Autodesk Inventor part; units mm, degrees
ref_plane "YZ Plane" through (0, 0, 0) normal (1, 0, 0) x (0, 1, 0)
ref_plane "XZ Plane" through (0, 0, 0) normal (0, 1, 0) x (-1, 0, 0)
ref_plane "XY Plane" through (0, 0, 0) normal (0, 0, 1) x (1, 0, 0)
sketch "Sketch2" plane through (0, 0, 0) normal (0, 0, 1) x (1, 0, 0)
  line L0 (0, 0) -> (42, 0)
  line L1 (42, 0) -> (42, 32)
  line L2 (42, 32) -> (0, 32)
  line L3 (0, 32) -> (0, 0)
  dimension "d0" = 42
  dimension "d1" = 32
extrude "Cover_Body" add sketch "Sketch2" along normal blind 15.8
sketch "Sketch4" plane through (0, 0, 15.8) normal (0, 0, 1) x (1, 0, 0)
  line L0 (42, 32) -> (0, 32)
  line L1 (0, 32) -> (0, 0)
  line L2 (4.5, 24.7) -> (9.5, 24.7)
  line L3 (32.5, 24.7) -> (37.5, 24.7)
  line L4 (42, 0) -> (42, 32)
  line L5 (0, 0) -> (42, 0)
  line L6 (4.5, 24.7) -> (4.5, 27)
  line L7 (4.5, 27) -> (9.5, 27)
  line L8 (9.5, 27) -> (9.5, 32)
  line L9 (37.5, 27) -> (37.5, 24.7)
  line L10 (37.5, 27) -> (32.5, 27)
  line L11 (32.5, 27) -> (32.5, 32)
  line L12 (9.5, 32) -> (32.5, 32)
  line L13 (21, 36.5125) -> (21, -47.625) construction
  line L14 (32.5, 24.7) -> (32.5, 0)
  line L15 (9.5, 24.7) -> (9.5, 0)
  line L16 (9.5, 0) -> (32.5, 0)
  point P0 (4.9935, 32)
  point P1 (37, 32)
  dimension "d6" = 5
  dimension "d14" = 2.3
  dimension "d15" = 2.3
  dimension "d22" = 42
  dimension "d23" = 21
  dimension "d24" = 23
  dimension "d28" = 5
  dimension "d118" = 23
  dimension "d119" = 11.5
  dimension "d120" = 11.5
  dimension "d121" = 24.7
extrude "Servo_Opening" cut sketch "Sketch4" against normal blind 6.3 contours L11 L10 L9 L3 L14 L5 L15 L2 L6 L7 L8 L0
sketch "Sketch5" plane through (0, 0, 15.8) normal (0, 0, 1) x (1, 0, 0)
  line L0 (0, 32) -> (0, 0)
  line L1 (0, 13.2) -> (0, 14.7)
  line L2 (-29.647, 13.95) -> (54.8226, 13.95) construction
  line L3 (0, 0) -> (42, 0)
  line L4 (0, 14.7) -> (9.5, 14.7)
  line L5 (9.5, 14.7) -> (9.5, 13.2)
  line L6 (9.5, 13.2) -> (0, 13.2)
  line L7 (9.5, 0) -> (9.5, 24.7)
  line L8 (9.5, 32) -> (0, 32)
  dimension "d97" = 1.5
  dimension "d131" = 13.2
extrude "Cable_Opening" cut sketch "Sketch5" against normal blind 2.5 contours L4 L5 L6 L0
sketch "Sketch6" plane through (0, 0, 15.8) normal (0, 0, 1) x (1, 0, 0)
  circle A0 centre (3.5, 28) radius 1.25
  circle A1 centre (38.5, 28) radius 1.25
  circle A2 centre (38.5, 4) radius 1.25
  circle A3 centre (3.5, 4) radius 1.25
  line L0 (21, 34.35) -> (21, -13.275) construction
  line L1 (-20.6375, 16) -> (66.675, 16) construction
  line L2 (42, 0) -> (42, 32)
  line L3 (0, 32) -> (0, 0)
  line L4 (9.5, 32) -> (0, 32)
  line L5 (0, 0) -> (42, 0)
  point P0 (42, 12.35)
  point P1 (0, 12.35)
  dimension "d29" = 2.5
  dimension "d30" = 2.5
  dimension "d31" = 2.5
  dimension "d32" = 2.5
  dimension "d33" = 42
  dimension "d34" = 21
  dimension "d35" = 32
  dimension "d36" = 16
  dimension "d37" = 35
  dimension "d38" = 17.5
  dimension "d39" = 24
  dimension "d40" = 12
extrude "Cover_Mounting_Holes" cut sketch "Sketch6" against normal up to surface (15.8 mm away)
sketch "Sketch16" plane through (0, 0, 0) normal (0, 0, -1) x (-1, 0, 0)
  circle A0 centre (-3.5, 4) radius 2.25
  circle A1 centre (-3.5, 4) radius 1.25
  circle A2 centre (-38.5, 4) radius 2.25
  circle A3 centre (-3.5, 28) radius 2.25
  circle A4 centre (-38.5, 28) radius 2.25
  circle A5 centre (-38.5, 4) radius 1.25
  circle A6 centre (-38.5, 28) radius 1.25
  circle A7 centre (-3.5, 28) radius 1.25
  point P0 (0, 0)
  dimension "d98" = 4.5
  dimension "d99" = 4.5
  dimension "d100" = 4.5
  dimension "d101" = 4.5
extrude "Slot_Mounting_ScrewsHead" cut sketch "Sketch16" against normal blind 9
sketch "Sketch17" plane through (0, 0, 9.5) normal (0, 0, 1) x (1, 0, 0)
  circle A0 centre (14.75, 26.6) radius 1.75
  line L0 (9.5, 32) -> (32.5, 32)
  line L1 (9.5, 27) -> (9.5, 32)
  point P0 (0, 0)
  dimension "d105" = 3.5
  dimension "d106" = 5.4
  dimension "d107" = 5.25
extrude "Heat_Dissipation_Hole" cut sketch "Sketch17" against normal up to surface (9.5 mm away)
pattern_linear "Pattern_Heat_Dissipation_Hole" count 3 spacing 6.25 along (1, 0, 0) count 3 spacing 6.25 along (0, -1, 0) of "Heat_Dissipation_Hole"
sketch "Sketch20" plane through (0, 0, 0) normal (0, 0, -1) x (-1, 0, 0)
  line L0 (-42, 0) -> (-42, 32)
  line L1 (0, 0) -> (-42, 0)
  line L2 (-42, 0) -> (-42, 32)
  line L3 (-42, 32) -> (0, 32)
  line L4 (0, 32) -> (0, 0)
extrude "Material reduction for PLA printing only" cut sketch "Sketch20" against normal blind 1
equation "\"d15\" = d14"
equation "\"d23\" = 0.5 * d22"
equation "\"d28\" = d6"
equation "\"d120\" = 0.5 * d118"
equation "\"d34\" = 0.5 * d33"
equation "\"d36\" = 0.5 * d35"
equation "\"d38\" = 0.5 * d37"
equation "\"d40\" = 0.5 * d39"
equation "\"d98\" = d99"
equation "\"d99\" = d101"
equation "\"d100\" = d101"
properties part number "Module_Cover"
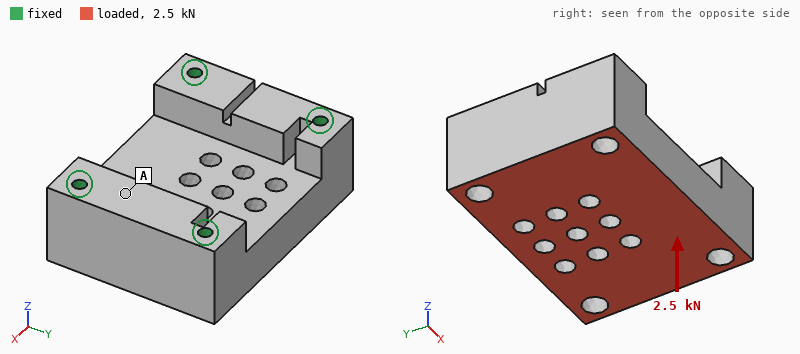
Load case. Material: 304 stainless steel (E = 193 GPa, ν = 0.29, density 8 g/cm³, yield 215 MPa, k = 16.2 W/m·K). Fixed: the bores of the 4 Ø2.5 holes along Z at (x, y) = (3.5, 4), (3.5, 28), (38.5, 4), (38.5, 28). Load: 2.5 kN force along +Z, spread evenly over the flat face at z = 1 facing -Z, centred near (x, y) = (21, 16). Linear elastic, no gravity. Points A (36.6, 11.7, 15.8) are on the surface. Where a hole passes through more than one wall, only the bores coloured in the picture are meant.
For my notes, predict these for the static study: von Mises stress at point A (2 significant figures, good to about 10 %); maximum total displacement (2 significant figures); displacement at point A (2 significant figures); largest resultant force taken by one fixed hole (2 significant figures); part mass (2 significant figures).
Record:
4.0 MPa
1.9 µm
0.81 µm
770 N
110 g
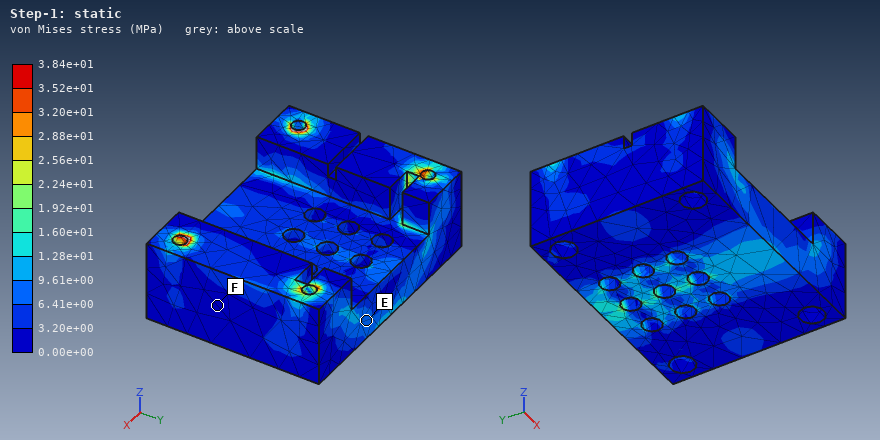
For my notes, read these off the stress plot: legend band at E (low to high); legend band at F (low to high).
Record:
6.41e+00 to 9.61e+00 MPa
0.00e+00 to 3.20e+00 MPa
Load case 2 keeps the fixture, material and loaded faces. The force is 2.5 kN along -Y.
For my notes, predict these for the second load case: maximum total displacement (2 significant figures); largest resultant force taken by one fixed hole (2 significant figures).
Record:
2.2 µm
880 N
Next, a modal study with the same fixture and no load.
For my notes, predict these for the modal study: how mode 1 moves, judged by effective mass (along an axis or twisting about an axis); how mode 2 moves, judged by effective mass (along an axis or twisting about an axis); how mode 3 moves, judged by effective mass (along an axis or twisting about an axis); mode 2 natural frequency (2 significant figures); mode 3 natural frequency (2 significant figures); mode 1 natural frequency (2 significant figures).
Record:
along Z
along X
along Y
25 kHz
27 kHz
22 kHz
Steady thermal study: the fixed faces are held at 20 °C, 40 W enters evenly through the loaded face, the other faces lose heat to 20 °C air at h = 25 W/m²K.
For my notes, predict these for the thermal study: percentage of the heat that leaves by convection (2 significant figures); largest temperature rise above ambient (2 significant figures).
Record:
12 %
71 K
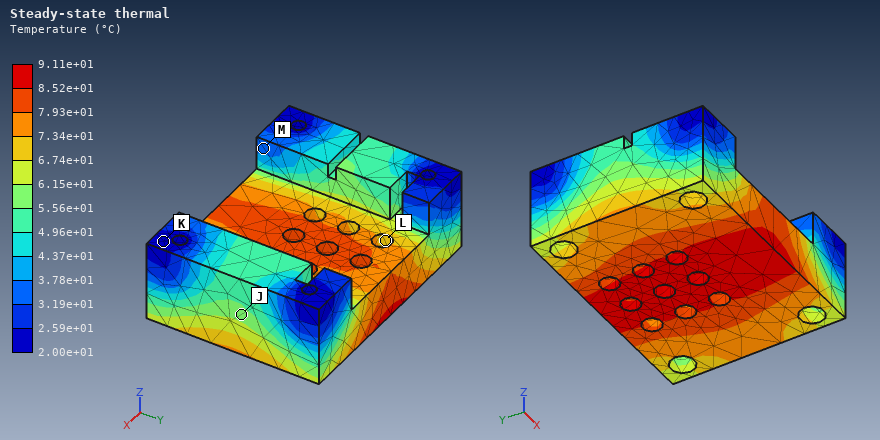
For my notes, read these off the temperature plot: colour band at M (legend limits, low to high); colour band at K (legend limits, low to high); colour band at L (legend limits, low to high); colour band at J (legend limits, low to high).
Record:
3.19e+01 to 3.78e+01 °C
2.00e+01 to 2.59e+01 °C
6.74e+01 to 7.34e+01 °C
5.56e+01 to 6.15e+01 °C
